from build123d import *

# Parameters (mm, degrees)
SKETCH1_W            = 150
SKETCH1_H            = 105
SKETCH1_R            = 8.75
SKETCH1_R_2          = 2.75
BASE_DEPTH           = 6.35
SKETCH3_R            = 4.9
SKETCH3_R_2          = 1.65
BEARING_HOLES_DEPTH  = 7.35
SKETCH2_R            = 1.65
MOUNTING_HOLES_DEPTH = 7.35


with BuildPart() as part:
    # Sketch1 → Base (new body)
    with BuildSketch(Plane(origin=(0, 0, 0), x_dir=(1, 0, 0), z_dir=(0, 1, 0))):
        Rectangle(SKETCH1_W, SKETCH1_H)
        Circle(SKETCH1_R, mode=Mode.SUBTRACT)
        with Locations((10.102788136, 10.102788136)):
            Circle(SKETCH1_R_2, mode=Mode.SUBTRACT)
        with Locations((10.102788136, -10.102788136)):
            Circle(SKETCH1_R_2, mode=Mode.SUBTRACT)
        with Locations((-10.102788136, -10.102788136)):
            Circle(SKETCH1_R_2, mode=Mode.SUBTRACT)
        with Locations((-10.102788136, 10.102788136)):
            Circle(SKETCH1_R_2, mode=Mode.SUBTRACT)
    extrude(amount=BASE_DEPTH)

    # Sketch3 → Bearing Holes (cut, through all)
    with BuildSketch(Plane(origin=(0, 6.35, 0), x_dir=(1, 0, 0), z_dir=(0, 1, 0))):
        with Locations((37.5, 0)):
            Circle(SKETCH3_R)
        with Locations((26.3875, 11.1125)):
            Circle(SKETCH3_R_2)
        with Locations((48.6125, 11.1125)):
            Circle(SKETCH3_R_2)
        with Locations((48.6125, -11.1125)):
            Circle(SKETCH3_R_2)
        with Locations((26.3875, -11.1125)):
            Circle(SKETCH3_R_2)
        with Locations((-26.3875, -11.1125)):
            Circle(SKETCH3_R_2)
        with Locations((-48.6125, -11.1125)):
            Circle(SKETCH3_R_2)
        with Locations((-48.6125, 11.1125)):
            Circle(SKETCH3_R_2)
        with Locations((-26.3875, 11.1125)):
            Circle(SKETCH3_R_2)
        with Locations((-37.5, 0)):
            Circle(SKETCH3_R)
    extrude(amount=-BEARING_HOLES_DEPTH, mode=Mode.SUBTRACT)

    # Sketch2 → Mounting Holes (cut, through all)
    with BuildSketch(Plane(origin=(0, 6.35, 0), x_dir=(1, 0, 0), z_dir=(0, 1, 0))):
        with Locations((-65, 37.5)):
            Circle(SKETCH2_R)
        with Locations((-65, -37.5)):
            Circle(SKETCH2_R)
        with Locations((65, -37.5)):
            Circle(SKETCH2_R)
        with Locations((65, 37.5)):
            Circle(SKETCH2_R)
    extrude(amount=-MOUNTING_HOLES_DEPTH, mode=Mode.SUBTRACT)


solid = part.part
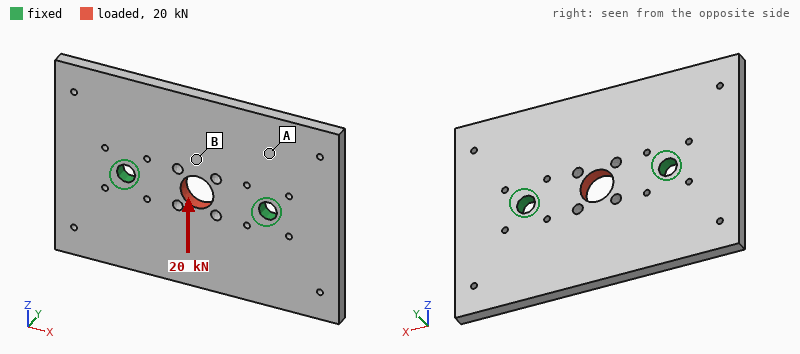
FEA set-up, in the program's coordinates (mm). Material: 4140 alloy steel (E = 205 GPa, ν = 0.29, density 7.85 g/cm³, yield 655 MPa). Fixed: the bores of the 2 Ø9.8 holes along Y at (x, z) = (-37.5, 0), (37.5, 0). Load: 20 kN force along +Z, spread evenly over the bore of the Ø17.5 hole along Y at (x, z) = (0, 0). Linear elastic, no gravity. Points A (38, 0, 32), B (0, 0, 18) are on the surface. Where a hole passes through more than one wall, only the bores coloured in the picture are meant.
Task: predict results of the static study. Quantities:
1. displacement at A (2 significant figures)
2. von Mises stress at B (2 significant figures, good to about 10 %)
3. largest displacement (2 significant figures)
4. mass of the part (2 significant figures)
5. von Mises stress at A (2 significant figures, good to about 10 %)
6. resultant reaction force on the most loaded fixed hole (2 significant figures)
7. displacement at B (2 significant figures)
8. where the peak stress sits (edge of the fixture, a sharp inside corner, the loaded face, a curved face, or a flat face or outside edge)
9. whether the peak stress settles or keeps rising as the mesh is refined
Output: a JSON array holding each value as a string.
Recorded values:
["3.4 µm", "43 MPa", "14 µm", "760 g", "14 MPa", "10 kN", "11 µm", "edge of the fixture", "keeps rising"]
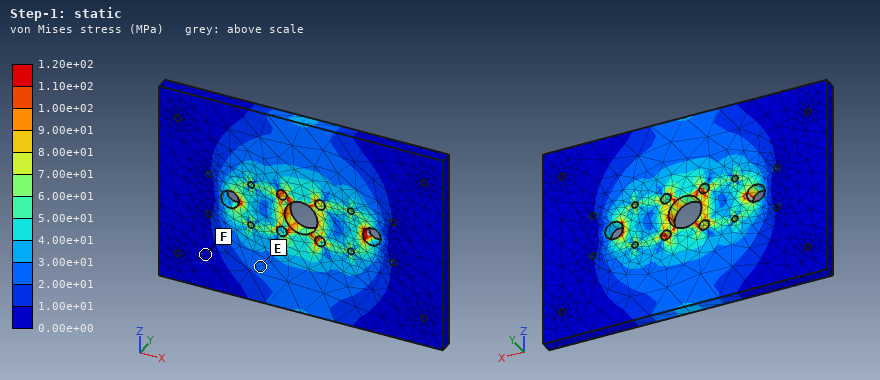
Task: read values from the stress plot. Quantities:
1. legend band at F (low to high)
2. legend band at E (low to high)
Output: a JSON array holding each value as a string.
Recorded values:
["0.00e+00 to 1.00e+01 MPa", "2.00e+01 to 3.00e+01 MPa"]
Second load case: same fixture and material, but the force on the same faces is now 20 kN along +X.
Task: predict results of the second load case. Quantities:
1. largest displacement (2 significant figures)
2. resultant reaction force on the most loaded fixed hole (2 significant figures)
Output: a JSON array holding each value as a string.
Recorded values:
["10 µm", "10 kN"]
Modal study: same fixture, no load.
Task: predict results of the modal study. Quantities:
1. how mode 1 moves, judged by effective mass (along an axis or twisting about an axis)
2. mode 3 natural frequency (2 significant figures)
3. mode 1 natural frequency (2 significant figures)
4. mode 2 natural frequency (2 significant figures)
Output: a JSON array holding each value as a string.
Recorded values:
["twisting about X", "2000 Hz", "1500 Hz", "1900 Hz"]
